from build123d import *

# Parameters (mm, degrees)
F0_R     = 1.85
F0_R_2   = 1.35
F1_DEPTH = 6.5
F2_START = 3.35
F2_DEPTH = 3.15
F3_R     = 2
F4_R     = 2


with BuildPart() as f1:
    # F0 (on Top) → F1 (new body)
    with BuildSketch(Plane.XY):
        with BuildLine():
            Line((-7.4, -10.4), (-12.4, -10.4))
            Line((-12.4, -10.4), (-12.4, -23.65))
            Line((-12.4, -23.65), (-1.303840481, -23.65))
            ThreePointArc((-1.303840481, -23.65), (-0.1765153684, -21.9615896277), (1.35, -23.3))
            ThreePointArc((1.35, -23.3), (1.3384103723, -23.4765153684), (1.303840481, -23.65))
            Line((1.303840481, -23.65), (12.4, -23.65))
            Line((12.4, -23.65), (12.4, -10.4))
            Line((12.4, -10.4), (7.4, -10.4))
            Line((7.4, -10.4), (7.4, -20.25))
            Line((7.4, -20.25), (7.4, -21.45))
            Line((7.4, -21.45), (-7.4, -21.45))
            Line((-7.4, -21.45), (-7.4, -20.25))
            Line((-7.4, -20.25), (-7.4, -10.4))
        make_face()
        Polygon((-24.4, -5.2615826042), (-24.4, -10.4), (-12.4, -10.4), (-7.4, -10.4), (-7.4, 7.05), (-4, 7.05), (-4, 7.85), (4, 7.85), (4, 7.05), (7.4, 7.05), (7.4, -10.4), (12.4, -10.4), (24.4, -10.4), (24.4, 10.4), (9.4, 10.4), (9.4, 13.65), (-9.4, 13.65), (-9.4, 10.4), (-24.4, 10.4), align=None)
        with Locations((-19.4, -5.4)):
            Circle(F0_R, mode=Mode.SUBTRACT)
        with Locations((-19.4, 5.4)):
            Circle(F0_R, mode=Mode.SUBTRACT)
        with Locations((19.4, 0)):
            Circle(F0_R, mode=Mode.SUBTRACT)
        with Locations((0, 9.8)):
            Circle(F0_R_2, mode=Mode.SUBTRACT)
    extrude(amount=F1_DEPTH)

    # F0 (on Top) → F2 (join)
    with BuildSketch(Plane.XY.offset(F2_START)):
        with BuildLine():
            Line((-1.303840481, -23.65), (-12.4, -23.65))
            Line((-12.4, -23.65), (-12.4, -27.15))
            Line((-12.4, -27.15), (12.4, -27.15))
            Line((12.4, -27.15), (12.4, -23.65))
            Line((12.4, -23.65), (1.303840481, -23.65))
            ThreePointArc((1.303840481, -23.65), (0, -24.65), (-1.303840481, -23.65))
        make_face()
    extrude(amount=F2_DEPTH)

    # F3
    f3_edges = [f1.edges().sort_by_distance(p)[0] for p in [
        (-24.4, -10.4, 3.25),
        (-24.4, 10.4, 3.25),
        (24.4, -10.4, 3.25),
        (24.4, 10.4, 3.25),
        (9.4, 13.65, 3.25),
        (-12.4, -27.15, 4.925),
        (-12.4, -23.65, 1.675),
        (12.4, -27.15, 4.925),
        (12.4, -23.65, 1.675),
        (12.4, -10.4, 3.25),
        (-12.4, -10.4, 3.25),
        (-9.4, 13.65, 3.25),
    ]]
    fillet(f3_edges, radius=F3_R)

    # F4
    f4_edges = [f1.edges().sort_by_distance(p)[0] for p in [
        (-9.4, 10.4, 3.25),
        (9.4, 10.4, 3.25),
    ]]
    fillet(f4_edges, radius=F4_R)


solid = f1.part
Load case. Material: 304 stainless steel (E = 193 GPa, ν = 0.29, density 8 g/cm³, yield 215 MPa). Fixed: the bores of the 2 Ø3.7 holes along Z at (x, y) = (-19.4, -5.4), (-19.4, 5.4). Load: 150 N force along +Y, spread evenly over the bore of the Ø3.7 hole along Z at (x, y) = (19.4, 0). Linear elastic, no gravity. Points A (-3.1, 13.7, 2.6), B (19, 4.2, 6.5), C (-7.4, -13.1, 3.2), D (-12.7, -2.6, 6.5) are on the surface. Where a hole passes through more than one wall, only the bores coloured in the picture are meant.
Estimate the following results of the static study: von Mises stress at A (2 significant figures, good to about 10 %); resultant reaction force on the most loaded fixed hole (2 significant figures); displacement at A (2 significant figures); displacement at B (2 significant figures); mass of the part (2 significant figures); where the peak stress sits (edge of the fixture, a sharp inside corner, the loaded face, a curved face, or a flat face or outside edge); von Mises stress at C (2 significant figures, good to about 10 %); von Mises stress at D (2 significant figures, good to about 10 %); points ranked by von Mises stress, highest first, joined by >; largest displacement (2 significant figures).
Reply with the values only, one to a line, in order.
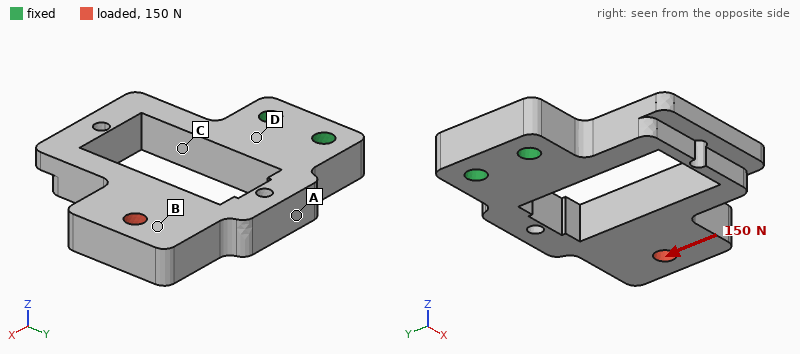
21 MPa
430 N
6.0 µm
19 µm
51 g
a curved face
35 MPa
11 MPa
C > A > D > B
22 µm
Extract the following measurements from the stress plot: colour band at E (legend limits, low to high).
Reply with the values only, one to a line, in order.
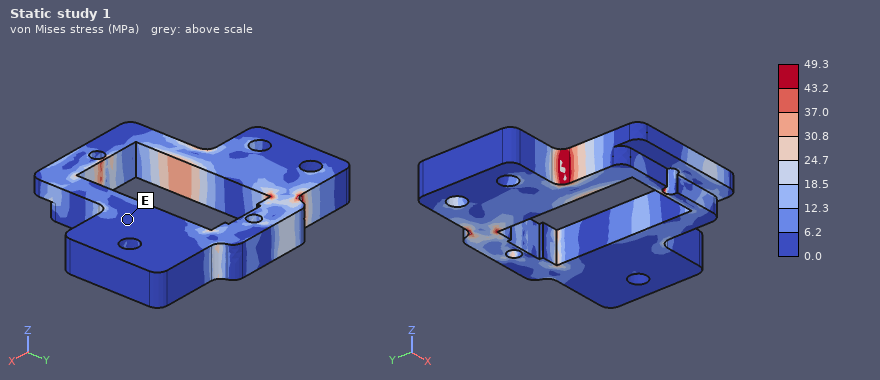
0.0 to 6.2 MPa
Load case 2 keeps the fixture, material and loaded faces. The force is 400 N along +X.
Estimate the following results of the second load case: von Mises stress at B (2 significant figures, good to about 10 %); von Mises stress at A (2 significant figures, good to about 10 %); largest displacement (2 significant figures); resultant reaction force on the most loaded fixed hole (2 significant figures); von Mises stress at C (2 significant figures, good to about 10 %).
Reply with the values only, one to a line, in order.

5.7 MPa
7.1 MPa
15 µm
220 N
31 MPa
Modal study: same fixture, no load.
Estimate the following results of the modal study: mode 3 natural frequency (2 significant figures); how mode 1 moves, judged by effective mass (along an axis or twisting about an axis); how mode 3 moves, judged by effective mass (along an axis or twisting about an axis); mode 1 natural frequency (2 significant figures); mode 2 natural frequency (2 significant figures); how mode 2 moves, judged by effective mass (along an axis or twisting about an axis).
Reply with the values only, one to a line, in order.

4500 Hz
along Z
twisting about X
1700 Hz
3000 Hz
along Y
